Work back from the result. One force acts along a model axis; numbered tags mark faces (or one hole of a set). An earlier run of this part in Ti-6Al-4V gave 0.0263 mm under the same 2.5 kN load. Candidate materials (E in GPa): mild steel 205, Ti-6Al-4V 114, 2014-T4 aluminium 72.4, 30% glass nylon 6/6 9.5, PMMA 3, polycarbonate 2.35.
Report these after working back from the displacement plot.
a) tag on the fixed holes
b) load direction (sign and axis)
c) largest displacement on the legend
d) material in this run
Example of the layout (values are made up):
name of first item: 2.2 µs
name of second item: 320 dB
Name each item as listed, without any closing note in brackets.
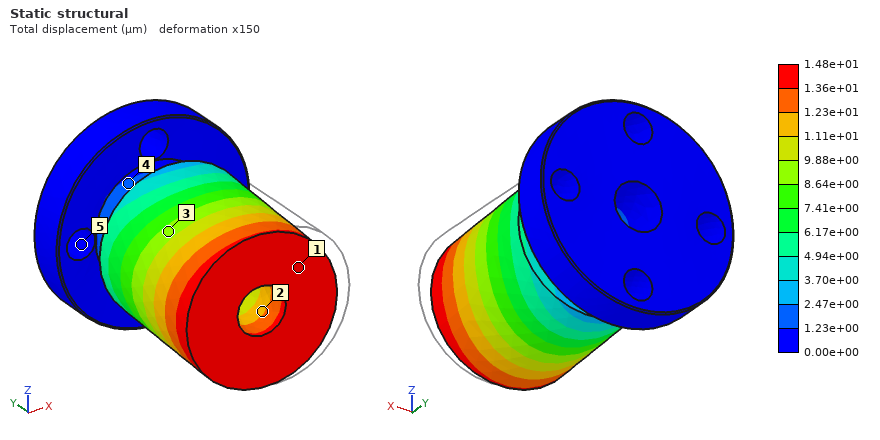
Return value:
tag on the fixed holes: 5
load direction: -X
largest displacement on the legend: 1.48e+01 µm
material in this run: mild steel
